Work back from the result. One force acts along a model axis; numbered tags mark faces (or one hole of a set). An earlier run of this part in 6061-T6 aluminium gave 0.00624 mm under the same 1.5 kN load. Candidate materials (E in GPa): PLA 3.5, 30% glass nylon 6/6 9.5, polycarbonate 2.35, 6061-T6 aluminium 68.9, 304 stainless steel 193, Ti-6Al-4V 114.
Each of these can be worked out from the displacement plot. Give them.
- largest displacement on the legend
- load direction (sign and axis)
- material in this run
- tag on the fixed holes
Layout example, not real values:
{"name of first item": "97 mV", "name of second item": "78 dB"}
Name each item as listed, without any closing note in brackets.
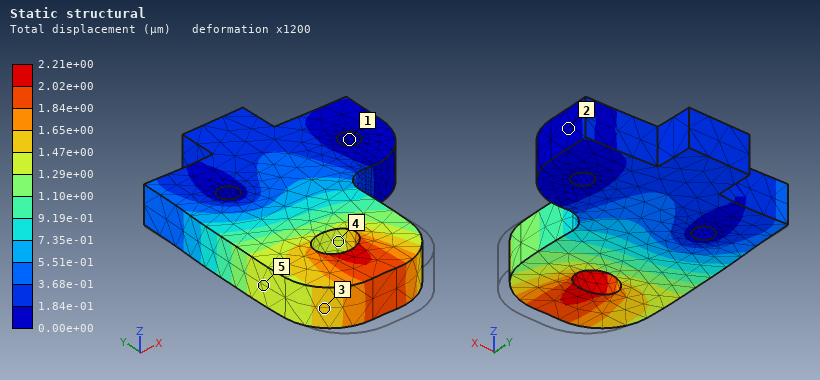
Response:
{"largest displacement on the legend": "2.21e+00 µm", "load direction": "+Y", "material in this run": "304 stainless steel", "tag on the fixed holes": "1"}
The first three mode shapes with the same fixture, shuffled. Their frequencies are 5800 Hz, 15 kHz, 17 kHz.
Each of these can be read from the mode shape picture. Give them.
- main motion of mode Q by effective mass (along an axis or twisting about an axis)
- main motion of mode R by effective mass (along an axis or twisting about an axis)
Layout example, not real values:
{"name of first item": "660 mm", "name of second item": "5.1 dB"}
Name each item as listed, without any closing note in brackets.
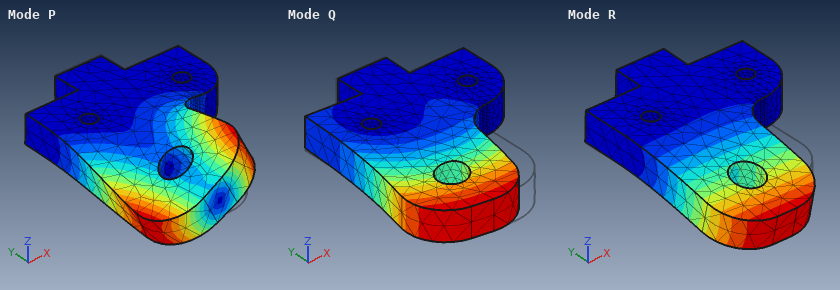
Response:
{"main motion of mode Q by effective mass": "along X", "main motion of mode R by effective mass": "along Z"}
